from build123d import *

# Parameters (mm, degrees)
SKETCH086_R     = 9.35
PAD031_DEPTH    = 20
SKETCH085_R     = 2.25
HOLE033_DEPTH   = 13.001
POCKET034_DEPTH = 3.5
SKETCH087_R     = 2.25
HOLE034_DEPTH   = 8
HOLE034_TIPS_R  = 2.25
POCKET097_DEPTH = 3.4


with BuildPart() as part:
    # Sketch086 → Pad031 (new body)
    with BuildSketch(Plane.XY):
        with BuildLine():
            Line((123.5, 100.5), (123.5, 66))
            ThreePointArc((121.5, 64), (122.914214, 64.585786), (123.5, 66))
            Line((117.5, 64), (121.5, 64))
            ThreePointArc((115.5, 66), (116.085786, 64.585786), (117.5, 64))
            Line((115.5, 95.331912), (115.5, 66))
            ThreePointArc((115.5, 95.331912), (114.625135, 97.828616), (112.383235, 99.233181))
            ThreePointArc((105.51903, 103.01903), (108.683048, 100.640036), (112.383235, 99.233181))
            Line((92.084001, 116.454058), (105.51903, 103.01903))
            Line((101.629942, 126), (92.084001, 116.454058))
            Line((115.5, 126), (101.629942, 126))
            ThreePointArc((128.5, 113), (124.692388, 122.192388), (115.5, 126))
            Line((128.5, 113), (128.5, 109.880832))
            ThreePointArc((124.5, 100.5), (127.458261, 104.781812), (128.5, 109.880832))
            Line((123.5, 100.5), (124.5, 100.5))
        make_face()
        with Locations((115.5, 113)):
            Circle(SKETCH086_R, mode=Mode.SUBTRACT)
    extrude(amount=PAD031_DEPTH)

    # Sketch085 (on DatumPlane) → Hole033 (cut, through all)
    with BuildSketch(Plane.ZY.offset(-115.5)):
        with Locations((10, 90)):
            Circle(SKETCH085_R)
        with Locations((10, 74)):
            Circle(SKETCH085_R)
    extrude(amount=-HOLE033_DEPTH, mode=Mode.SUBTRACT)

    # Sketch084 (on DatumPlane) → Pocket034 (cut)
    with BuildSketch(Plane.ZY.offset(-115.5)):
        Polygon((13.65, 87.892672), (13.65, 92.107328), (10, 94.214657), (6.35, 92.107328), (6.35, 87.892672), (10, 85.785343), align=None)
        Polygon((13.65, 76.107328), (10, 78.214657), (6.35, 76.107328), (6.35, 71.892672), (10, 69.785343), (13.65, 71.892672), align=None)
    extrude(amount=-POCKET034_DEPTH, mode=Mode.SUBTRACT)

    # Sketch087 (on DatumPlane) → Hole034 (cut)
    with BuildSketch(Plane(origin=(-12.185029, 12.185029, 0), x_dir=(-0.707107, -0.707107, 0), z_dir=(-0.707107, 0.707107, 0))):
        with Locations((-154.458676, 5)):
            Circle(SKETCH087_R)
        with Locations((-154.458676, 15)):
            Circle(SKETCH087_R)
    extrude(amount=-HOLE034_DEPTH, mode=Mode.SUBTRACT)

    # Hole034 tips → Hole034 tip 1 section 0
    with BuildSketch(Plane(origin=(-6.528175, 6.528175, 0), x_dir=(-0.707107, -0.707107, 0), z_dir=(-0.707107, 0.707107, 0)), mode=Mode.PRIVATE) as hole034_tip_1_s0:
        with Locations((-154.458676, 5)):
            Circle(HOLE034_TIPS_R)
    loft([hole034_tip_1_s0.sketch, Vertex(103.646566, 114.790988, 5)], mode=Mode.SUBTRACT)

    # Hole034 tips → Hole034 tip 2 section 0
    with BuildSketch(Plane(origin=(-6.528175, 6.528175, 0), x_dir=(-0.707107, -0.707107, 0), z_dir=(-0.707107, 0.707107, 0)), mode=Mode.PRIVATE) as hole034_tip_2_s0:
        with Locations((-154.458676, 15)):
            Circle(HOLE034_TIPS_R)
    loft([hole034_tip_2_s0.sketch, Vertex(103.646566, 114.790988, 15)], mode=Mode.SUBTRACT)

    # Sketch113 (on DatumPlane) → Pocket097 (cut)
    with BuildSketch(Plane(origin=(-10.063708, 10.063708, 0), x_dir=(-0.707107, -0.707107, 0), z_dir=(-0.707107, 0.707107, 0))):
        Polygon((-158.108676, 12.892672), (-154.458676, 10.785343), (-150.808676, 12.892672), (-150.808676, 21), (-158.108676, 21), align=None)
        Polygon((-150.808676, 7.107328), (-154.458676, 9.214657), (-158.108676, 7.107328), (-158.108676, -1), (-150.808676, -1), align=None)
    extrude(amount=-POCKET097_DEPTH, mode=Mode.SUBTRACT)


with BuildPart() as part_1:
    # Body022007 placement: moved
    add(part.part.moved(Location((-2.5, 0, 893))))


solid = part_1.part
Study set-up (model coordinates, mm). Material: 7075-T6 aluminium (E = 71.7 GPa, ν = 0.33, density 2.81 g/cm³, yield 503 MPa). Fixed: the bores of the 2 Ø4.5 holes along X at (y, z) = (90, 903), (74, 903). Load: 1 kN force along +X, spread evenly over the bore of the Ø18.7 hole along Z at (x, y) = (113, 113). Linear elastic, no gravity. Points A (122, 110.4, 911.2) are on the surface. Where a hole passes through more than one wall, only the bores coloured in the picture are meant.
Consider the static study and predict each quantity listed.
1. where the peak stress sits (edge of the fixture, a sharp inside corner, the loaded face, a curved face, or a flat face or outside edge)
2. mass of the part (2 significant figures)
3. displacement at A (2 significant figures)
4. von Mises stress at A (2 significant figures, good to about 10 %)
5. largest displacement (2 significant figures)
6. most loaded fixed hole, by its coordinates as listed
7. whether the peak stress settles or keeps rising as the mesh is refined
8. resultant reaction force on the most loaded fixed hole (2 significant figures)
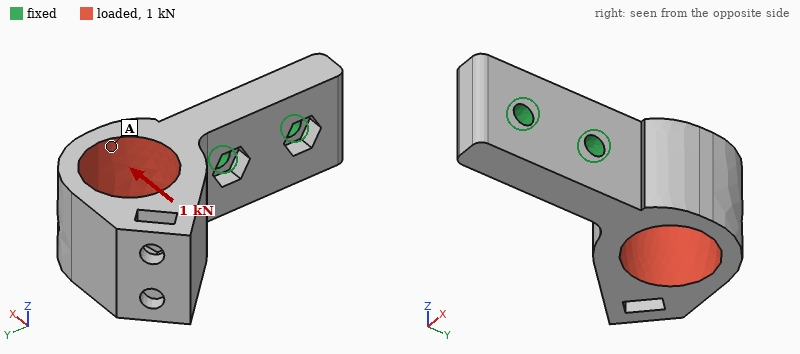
edge of the fixture
38 g
0.096 mm
22 MPa
0.22 mm
(90, 903)
keeps rising
2.0 kN
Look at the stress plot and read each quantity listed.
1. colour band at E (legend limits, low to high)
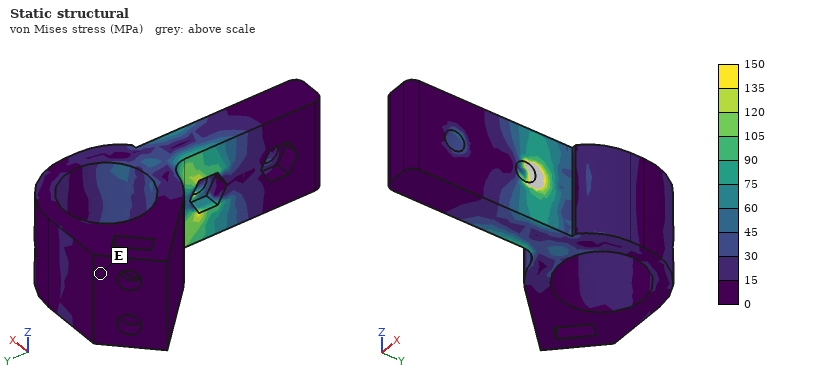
0 to 15 MPa
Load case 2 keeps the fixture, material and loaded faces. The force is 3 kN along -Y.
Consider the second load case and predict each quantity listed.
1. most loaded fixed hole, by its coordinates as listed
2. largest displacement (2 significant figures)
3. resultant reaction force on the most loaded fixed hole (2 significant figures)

(90, 903)
0.16 mm
1.8 kN
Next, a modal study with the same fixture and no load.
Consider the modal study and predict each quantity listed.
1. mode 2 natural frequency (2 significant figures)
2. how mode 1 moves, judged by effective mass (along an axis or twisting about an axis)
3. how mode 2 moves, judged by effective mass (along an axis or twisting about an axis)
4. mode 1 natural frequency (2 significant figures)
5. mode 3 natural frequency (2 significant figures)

3700 Hz
along X
along Z
2400 Hz
7300 Hz
